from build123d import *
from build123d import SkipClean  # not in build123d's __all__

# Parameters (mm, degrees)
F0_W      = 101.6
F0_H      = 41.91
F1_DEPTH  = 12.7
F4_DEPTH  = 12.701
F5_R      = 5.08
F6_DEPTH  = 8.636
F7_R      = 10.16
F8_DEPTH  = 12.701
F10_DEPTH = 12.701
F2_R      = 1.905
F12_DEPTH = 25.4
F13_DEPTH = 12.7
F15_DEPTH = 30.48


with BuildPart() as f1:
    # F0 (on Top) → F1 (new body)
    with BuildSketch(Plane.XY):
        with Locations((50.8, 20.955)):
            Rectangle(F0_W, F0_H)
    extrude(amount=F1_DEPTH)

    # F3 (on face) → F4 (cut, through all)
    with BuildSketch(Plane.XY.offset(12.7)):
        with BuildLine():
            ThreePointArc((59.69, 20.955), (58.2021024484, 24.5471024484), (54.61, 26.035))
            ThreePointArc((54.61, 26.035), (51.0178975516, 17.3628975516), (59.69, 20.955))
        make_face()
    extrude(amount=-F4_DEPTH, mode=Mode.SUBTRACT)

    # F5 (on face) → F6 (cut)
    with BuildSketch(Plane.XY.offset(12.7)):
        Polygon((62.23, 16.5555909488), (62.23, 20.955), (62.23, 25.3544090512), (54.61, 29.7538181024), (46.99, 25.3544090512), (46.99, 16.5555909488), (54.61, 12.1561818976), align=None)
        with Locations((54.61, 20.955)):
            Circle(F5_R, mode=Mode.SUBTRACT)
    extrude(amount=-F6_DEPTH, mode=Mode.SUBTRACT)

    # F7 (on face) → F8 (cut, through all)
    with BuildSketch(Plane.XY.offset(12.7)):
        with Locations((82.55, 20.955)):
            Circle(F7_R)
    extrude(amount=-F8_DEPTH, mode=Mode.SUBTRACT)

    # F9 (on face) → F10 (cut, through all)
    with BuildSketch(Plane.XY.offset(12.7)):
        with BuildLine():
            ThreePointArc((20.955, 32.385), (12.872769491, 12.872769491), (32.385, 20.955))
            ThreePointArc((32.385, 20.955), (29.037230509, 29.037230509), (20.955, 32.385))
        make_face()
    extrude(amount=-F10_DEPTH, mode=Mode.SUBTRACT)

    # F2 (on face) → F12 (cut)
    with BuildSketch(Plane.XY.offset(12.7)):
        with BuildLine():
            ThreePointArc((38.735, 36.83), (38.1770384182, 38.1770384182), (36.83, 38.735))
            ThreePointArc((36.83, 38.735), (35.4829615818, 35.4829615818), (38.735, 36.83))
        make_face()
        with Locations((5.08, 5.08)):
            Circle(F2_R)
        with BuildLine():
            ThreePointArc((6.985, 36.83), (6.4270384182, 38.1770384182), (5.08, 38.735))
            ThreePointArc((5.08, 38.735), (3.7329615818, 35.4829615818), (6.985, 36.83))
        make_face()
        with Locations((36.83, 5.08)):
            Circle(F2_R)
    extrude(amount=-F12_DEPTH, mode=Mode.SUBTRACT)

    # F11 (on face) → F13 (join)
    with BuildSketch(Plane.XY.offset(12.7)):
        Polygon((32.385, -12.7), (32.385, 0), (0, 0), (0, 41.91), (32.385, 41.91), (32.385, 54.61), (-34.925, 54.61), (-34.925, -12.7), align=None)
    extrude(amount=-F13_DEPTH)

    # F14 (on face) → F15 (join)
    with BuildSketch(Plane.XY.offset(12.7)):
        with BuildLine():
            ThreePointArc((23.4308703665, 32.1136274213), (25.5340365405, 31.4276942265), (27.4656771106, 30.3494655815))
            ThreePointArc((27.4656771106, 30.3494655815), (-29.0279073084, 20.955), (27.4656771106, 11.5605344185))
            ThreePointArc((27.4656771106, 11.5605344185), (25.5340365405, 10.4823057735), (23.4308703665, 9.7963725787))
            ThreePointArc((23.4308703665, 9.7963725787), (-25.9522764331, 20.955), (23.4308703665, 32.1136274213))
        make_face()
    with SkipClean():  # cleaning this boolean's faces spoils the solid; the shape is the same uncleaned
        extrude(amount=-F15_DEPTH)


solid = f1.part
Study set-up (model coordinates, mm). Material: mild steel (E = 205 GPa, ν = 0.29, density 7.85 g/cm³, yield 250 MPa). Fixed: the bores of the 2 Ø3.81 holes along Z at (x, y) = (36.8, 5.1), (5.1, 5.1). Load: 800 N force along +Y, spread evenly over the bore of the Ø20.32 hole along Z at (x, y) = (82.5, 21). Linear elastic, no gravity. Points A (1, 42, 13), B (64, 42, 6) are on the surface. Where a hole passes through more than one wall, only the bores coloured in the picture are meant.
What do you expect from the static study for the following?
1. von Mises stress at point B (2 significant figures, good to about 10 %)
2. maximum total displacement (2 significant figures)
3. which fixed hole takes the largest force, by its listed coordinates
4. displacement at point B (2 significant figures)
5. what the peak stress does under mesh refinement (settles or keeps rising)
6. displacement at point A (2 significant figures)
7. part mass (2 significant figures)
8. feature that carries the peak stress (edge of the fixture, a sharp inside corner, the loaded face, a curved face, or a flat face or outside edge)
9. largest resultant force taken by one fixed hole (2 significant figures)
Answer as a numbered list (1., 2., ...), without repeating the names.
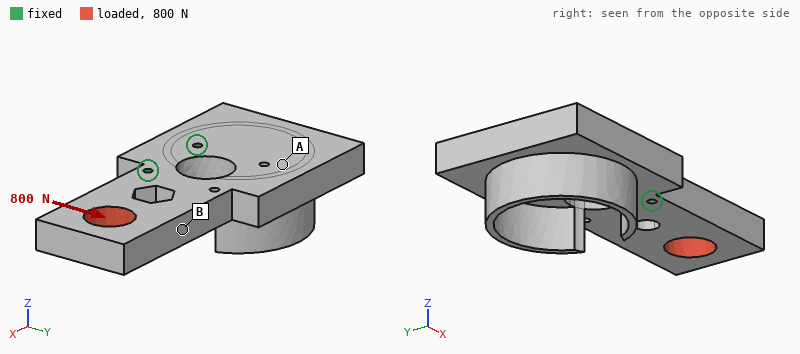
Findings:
1. 4.5 MPa
2. 15 µm
3. (36.8, 5.1)
4. 7.6 µm
5. keeps rising
6. 3.2 µm
7. 710 g
8. edge of the fixture
9. 1.9 kN
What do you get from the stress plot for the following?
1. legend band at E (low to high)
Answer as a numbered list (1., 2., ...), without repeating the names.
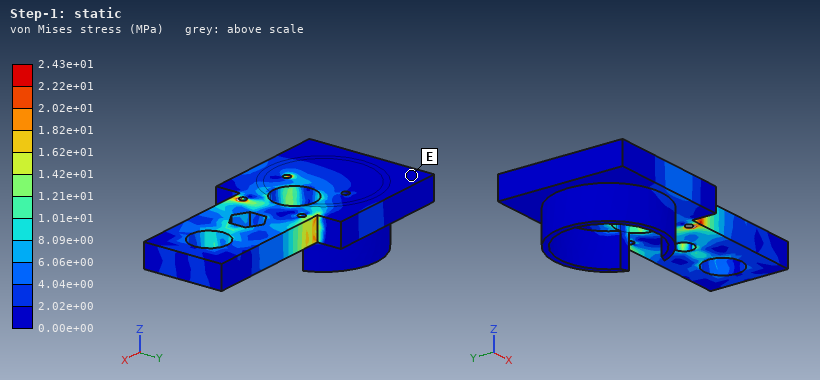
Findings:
1. 0.00e+00 to 2.02e+00 MPa
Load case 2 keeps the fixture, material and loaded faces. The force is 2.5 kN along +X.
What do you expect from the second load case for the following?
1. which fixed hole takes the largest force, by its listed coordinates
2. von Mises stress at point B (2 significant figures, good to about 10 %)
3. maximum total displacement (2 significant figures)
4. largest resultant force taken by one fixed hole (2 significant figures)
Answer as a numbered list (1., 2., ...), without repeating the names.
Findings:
1. (36.8, 5.1)
2. 7.1 MPa
3. 9.9 µm
4. 1.8 kN
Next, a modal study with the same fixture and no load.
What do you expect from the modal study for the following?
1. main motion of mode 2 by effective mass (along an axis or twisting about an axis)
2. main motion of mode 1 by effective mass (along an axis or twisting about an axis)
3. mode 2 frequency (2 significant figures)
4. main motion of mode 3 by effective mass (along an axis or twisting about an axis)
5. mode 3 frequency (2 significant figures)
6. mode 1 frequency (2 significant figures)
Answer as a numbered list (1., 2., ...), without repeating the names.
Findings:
1. along Z
2. along Z
3. 2400 Hz
4. along X
5. 3100 Hz
6. 1900 Hz
